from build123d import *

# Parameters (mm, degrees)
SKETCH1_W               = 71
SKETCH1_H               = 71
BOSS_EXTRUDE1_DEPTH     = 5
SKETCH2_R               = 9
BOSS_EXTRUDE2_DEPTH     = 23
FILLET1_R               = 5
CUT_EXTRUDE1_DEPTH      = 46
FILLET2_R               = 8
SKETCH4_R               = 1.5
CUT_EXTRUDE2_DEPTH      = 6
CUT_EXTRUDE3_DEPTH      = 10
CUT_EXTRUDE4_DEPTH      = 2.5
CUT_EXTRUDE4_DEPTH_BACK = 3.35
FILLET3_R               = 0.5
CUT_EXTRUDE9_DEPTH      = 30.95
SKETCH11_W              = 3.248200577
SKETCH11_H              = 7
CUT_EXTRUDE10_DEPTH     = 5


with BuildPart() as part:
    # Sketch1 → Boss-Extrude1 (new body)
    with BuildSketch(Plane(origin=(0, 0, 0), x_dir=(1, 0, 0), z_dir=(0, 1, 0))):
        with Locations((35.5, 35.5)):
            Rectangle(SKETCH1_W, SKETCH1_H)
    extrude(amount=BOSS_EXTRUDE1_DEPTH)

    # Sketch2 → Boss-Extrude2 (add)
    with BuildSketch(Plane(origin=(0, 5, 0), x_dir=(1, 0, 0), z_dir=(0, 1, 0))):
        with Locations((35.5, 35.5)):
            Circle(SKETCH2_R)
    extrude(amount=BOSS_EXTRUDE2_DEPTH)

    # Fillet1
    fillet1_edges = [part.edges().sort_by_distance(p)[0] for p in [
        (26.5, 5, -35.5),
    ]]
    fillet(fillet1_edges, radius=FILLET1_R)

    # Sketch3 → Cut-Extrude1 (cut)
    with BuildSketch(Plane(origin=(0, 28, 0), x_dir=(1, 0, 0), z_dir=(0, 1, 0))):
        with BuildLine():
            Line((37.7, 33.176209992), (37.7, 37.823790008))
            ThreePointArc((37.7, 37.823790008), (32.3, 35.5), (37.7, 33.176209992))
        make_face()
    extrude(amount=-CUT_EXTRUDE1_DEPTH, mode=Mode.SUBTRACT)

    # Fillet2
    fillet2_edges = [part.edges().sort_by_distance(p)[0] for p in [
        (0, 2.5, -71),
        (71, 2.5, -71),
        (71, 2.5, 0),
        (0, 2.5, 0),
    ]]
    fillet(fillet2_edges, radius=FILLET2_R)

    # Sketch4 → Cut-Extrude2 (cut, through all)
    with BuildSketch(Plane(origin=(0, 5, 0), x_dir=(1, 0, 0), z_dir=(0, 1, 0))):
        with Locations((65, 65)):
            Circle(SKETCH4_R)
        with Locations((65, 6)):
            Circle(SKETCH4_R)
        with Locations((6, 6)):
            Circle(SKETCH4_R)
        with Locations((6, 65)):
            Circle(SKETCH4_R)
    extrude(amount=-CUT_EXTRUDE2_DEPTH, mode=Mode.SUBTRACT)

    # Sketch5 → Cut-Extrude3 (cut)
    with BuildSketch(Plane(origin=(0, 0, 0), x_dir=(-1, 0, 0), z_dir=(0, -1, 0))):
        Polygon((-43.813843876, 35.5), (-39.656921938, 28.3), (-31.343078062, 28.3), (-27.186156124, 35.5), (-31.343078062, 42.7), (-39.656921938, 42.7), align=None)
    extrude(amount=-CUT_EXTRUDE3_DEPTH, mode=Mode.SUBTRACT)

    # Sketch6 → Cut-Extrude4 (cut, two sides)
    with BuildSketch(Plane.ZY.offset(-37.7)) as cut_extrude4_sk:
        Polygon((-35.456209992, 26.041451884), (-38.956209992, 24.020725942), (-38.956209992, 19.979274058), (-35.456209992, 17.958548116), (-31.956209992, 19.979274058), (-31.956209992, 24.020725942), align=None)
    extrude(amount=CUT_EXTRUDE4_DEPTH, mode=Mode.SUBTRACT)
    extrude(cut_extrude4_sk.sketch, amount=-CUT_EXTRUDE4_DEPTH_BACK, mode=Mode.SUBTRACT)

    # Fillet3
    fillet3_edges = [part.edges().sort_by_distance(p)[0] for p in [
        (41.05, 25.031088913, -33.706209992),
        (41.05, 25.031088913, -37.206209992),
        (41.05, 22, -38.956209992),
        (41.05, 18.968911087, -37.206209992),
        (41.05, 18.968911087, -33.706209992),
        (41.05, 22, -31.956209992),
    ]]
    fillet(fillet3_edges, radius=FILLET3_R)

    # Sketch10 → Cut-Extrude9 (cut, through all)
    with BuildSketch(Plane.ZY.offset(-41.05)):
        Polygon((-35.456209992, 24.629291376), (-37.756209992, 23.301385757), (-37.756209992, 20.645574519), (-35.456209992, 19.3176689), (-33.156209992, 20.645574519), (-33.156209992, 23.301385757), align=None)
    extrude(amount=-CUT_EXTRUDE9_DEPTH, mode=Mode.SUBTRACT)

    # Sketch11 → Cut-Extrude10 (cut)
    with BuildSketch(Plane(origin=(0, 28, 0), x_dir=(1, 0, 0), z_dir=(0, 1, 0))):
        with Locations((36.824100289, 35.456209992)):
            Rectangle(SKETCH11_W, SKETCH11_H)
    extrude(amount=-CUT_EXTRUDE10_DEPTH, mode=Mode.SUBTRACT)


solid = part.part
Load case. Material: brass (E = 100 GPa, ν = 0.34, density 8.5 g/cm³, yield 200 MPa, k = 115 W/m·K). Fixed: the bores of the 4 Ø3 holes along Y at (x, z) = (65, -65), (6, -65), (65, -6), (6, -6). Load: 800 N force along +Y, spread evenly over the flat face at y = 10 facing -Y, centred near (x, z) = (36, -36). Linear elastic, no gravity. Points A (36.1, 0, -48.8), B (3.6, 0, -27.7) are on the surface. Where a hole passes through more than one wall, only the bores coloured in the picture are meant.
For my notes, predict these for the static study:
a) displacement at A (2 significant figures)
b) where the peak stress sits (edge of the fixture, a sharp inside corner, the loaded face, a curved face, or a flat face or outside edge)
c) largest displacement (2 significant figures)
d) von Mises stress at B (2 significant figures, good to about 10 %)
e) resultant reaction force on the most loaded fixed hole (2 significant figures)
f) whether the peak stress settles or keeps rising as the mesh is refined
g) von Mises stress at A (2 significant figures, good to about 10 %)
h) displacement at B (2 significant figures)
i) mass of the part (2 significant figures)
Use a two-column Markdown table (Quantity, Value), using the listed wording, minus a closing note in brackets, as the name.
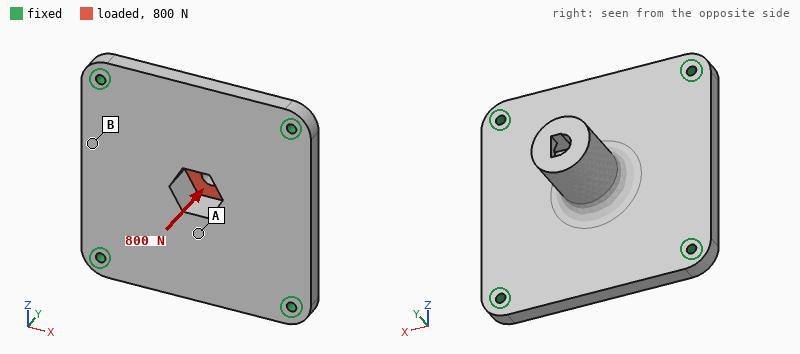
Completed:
| Quantity | Value |
|---|---|
| displacement at A | 25 µm |
| where the peak stress sits | edge of the fixture |
| largest displacement | 28 µm |
| von Mises stress at B | 9.5 MPa |
| resultant reaction force on the most loaded fixed hole | 210 N |
| whether the peak stress settles or keeps rising as the mesh is refined | keeps rising |
| von Mises stress at A | 19 MPa |
| displacement at B | 9.0 µm |
| mass of the part | 240 g |
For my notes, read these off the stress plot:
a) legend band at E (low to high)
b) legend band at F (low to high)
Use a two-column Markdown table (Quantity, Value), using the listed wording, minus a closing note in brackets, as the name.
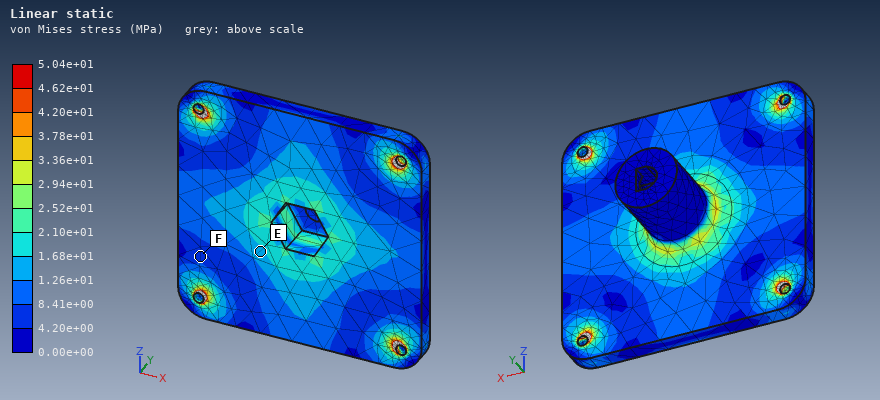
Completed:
| Quantity | Value |
|---|---|
| legend band at E | 1.26e+01 to 1.68e+01 MPa |
| legend band at F | 4.20e+00 to 8.41e+00 MPa |
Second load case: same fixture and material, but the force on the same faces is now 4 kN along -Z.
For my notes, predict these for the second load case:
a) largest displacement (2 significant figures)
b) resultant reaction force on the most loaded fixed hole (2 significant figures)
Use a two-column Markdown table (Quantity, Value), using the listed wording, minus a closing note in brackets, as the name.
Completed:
| Quantity | Value |
|---|---|
| largest displacement | 60 µm |
| resultant reaction force on the most loaded fixed hole | 1.2 kN |
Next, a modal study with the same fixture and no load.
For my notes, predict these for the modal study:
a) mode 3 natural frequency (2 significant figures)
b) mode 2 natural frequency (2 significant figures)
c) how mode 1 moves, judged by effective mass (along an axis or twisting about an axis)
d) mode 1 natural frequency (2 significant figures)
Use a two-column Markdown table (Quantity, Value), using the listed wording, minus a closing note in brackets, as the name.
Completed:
| Quantity | Value |
|---|---|
| mode 3 natural frequency | 4100 Hz |
| mode 2 natural frequency | 4000 Hz |
| how mode 1 moves, judged by effective mass | along Y |
| mode 1 natural frequency | 2700 Hz |
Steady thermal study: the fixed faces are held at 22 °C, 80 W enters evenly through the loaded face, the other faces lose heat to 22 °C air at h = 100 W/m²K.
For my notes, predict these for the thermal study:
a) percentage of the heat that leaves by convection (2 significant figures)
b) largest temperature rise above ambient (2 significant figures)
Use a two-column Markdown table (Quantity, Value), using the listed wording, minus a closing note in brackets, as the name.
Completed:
| Quantity | Value |
|---|---|
| percentage of the heat that leaves by convection | 40 % |
| largest temperature rise above ambient | 84 K |
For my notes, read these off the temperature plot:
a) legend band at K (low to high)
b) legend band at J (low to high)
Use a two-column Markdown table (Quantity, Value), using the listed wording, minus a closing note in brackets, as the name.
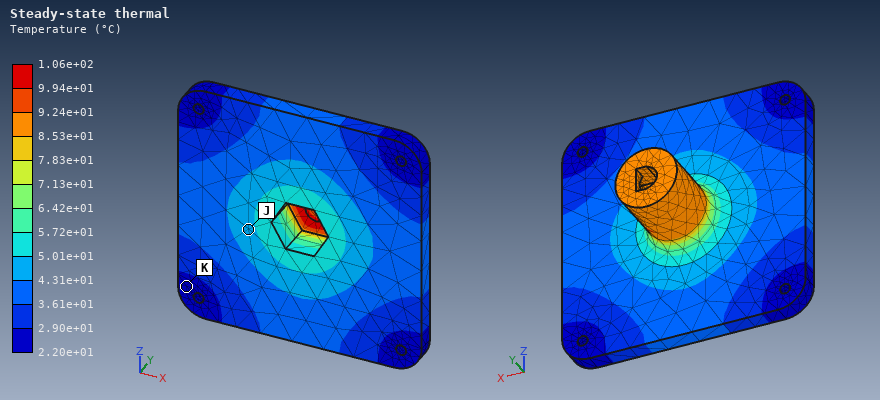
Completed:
| Quantity | Value |
|---|---|
| legend band at K | 2.20e+01 to 2.90e+01 °C |
| legend band at J | 4.31e+01 to 5.01e+01 °C |
